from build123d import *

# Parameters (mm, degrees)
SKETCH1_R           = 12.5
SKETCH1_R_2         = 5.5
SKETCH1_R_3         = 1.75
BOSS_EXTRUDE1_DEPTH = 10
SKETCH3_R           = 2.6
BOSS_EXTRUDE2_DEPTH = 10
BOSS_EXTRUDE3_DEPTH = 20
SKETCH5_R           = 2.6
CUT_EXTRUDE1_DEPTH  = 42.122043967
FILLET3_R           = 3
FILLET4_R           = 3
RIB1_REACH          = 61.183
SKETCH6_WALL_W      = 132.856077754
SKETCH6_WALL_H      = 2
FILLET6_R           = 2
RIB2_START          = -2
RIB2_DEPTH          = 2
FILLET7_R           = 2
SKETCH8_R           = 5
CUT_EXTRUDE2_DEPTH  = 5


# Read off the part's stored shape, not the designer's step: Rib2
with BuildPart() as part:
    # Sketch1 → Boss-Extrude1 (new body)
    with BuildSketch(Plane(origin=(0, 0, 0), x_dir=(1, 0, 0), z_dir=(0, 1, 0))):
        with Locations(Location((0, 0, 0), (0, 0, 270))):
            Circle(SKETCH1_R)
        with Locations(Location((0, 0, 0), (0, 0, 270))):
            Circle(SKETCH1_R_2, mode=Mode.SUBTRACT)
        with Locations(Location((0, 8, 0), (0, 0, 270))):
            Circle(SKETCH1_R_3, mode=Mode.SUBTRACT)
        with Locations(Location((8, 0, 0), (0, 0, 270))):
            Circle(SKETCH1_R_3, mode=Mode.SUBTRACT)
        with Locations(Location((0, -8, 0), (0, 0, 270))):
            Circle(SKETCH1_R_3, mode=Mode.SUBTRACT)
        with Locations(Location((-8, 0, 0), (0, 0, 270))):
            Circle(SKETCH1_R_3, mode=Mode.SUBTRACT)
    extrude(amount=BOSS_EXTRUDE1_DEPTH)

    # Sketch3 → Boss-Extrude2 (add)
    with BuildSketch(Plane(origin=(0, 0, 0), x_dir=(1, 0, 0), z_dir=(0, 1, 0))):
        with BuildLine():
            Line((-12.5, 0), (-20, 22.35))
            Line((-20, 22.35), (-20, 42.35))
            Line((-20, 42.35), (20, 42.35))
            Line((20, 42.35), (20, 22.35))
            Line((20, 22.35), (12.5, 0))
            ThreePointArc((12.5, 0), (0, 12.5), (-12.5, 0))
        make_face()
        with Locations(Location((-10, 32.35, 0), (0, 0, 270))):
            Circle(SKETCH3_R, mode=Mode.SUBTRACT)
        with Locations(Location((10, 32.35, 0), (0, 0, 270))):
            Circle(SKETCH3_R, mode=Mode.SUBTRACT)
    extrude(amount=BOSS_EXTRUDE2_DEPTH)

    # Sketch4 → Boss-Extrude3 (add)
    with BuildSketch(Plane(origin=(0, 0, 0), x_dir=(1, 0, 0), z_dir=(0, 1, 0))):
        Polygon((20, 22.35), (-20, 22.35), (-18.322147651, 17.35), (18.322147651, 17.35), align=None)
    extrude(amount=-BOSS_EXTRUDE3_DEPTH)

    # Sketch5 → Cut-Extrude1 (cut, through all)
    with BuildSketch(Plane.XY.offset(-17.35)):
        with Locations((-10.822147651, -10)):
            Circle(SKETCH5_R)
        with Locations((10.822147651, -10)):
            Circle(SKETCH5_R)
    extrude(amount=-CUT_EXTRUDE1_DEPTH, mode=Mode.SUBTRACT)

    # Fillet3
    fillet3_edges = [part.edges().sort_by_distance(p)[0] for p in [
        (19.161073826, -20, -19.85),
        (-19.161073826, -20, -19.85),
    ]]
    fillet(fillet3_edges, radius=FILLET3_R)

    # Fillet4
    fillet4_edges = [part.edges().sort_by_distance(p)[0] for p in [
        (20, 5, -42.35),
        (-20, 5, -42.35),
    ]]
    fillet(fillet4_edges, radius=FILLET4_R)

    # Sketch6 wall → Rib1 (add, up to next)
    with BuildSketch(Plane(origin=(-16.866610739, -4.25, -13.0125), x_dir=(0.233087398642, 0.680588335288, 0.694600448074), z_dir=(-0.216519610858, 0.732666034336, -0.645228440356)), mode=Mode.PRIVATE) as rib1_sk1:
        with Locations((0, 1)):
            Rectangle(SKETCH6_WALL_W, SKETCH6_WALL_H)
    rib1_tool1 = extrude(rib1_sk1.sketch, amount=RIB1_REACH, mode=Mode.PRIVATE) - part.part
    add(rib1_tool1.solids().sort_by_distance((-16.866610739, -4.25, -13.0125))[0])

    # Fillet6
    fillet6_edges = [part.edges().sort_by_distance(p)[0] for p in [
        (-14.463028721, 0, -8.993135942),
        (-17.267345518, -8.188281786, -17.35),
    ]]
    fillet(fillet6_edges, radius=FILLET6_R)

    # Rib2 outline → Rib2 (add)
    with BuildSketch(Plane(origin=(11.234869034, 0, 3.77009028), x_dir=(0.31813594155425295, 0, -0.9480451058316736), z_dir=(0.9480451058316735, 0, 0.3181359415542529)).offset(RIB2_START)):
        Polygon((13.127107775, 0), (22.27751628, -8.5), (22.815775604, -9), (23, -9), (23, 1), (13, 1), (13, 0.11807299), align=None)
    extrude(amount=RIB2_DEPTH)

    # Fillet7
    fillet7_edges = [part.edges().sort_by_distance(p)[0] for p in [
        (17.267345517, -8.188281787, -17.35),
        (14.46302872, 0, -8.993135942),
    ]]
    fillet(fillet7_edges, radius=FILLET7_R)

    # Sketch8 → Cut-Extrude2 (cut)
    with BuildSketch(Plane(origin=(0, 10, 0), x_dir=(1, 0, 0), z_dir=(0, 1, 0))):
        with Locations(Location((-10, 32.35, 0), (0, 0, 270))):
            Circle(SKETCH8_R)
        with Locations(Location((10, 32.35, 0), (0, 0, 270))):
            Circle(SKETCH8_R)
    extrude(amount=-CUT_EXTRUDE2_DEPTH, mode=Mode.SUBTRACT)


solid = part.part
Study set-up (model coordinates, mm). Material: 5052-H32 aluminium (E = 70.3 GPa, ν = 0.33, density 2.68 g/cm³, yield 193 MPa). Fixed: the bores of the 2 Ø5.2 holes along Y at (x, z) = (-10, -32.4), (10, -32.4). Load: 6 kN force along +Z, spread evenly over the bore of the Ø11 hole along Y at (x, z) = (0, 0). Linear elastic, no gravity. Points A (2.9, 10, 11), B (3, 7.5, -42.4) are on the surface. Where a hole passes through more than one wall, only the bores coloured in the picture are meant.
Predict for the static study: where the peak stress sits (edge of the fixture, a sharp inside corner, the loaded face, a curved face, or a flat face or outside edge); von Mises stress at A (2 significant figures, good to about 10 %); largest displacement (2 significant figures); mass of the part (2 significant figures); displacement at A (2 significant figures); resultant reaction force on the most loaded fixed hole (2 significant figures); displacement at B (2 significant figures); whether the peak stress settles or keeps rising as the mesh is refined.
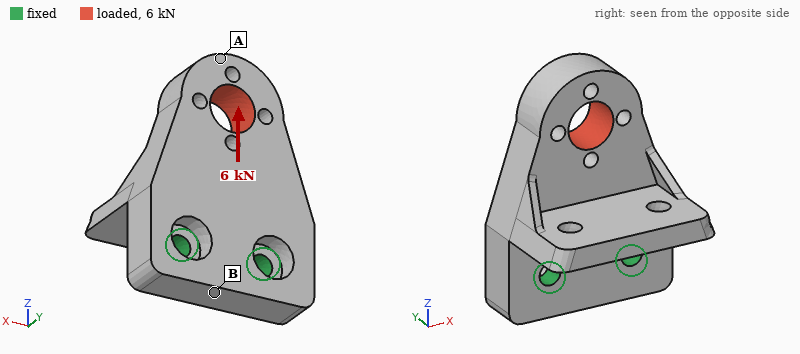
edge of the fixture
32 MPa
62 µm
51 g
60 µm
3.0 kN
11 µm
keeps rising
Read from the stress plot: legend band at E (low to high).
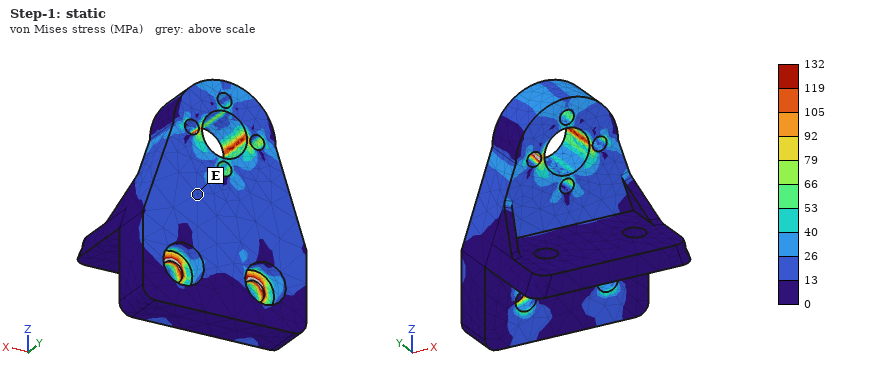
13 to 26 MPa
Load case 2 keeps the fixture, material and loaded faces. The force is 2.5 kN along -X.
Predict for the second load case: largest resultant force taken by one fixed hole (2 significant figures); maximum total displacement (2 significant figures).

3.7 kN
50 µm
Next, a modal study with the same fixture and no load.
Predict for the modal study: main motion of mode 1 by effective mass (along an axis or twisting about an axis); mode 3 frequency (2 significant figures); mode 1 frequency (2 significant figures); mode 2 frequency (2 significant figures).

along Y
10 kHz
3700 Hz
9700 Hz
